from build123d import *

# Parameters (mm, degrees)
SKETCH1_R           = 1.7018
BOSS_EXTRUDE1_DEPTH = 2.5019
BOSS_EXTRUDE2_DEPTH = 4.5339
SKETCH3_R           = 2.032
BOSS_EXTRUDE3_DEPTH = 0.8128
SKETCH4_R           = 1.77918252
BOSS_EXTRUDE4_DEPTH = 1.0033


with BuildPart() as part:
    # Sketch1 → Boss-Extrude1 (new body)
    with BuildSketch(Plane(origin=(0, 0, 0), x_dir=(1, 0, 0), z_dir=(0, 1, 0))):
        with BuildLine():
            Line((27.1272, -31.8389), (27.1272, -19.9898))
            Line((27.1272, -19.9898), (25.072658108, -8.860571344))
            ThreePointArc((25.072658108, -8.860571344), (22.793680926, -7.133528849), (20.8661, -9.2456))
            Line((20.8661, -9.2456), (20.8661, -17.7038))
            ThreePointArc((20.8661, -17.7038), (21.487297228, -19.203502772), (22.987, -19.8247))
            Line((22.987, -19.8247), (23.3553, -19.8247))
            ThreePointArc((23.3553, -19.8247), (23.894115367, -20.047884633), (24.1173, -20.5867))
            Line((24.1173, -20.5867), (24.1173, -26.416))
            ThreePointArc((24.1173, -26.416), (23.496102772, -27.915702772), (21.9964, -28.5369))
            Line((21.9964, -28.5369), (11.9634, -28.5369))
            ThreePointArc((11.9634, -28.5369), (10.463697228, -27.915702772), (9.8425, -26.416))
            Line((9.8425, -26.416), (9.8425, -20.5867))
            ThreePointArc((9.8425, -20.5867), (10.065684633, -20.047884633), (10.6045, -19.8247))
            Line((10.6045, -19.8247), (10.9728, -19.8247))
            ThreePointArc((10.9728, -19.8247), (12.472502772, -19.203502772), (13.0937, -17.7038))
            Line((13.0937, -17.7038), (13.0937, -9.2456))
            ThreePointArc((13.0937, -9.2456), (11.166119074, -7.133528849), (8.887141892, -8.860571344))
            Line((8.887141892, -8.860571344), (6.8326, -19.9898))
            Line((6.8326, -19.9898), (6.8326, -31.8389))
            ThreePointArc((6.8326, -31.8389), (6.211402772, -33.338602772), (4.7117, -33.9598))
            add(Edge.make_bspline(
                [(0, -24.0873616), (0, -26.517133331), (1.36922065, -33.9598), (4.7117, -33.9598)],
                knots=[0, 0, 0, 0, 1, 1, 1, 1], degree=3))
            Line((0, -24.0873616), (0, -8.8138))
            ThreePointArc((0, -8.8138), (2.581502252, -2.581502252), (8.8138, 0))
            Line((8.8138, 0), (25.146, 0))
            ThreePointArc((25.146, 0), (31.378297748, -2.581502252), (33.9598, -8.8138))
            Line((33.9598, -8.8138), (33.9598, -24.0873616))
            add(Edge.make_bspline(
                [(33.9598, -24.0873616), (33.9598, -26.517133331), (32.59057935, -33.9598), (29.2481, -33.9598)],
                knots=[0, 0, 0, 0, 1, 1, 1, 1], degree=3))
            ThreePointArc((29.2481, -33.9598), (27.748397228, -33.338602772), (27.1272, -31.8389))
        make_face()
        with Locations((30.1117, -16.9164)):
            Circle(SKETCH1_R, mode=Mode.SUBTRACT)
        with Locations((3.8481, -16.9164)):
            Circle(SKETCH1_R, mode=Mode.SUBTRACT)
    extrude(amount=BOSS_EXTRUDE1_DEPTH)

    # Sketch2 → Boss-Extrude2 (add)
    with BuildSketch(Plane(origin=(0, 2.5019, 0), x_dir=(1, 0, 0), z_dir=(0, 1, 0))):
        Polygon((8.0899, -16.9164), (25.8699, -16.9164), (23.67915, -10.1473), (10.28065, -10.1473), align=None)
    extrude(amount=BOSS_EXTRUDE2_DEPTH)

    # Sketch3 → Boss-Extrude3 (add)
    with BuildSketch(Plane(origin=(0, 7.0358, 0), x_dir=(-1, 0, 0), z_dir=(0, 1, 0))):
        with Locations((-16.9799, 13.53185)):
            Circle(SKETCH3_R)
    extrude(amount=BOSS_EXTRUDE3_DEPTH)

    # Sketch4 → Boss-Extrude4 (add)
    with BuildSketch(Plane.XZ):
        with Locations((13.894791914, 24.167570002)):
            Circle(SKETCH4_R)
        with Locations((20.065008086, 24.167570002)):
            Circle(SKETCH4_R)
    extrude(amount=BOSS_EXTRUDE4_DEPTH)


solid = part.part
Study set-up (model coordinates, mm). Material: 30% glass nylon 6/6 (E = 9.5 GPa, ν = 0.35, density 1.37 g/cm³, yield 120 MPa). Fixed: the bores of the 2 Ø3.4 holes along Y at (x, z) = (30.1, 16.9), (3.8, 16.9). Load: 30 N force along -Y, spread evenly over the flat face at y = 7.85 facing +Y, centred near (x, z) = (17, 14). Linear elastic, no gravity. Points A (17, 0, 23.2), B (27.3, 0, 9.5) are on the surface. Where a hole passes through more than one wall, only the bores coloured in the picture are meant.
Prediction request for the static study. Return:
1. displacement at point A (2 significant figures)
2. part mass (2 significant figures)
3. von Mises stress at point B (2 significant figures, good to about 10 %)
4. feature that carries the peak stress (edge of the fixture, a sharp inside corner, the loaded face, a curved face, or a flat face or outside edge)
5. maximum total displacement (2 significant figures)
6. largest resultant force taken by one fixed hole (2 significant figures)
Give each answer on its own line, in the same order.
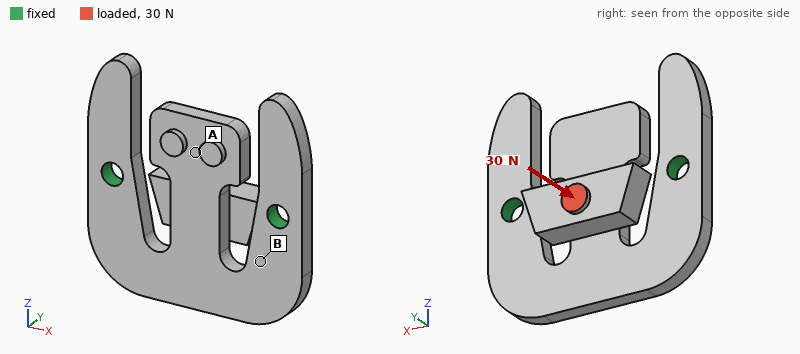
0.42 mm
3.4 g
12 MPa
a curved face
0.54 mm
15 N
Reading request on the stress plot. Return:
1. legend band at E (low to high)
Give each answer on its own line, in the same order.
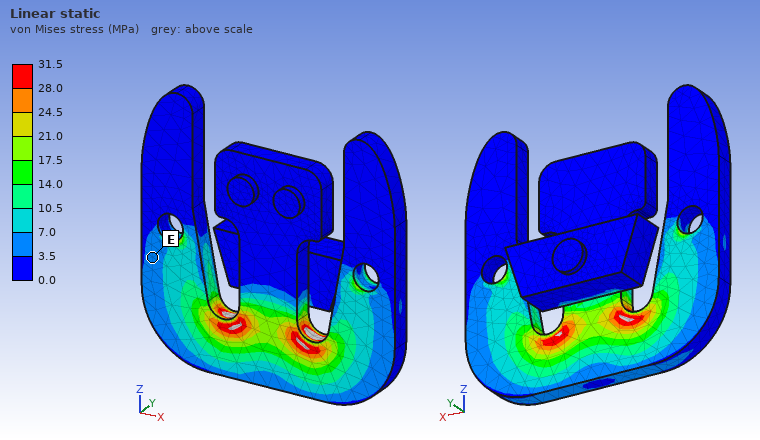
3.5 to 7.0 MPa
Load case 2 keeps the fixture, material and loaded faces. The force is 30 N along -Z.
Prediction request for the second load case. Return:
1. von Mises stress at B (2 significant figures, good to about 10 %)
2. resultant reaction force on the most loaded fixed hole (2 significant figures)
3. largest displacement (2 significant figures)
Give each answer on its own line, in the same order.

11 MPa
17 N
0.57 mm
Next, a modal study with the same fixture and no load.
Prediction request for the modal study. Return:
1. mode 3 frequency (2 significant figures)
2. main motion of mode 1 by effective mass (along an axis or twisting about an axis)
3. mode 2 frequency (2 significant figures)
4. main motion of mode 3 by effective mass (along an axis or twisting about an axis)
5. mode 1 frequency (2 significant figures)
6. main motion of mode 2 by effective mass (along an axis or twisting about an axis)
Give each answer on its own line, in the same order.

3200 Hz
along Y
2700 Hz
along X
970 Hz
along Y
